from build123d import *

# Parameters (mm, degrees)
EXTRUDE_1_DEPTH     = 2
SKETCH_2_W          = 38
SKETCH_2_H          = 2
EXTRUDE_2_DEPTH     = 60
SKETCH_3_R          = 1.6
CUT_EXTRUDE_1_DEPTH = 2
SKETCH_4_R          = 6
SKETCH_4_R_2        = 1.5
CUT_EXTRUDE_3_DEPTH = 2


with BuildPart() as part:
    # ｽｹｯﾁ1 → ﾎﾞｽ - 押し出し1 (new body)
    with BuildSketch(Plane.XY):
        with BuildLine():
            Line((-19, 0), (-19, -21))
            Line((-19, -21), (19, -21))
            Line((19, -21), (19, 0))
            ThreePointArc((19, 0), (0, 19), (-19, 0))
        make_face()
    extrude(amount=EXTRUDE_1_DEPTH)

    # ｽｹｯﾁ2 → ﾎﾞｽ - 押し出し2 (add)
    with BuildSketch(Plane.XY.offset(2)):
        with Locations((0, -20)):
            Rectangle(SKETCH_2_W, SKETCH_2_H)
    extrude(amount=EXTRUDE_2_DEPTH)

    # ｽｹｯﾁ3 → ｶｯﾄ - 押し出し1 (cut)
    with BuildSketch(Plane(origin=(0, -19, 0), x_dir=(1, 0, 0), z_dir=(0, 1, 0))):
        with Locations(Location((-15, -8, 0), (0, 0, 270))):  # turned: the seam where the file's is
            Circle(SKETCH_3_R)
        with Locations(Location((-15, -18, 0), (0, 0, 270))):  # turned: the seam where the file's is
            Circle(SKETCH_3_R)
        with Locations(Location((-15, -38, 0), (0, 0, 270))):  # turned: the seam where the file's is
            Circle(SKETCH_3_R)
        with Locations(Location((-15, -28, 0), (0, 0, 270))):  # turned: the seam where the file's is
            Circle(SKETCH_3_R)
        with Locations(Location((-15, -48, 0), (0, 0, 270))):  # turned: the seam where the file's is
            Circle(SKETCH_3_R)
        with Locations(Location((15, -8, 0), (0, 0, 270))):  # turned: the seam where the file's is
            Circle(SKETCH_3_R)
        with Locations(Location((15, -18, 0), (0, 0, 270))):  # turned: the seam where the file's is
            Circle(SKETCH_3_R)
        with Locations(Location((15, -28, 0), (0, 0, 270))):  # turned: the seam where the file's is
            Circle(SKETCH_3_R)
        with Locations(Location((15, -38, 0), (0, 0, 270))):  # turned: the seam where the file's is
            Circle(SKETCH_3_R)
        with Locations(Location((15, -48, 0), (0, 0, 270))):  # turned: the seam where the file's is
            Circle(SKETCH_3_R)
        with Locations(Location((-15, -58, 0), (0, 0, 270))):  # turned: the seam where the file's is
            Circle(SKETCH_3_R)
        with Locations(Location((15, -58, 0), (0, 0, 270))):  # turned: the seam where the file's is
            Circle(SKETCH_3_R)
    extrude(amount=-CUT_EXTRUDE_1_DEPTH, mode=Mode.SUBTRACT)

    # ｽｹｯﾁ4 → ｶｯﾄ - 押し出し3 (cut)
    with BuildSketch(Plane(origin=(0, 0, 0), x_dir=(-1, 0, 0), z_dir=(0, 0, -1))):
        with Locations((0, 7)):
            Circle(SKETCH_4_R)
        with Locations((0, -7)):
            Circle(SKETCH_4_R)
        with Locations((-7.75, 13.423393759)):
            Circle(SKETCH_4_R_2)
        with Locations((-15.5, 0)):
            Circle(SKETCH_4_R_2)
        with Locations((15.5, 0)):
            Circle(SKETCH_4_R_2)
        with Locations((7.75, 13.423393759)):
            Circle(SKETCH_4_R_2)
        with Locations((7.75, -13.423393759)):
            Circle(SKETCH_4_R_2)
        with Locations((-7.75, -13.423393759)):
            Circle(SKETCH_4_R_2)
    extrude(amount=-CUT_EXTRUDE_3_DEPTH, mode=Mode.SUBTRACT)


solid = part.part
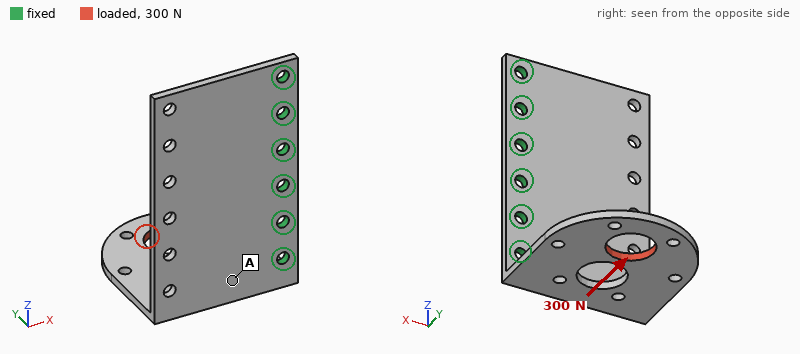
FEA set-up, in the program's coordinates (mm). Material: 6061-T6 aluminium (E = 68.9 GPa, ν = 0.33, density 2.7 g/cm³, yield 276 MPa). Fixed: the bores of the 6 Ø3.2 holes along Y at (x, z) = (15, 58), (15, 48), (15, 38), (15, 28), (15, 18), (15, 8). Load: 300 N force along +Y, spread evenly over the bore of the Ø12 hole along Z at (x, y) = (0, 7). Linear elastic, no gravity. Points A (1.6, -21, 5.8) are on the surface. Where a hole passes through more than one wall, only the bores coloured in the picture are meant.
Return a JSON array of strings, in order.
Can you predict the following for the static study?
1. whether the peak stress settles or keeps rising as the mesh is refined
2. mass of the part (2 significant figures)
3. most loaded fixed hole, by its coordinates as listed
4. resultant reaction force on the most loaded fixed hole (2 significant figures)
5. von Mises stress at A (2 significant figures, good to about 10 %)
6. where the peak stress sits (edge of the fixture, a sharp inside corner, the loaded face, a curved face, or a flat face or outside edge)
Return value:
["keeps rising", "18 g", "(15, 8)", "340 N", "38 MPa", "edge of the fixture"]
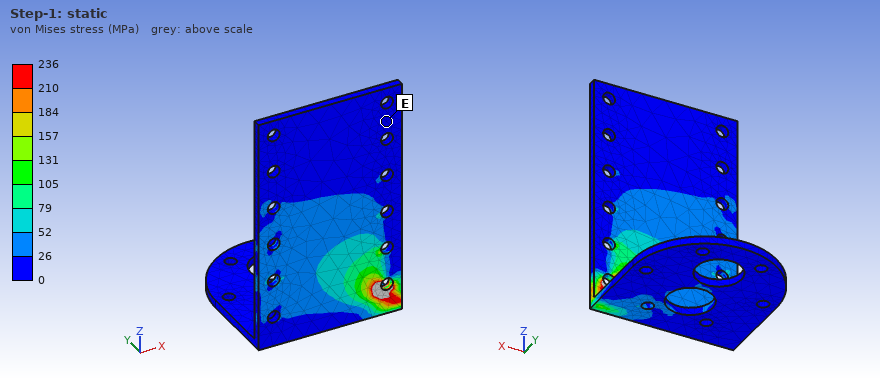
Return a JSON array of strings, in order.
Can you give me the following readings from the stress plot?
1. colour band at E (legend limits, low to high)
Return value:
["0 to 26 MPa"]
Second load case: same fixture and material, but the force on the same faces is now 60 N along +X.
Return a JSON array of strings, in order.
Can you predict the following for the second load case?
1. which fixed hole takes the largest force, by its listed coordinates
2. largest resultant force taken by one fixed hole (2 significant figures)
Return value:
["(15, 8)", "63 N"]
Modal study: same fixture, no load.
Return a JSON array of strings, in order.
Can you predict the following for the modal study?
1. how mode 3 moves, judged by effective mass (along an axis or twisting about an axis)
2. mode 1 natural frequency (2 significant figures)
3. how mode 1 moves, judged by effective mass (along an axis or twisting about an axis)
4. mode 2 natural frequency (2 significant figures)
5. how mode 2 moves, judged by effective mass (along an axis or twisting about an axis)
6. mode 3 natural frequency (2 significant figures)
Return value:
["along Y", "890 Hz", "along Z", "1200 Hz", "along Y", "2000 Hz"]
